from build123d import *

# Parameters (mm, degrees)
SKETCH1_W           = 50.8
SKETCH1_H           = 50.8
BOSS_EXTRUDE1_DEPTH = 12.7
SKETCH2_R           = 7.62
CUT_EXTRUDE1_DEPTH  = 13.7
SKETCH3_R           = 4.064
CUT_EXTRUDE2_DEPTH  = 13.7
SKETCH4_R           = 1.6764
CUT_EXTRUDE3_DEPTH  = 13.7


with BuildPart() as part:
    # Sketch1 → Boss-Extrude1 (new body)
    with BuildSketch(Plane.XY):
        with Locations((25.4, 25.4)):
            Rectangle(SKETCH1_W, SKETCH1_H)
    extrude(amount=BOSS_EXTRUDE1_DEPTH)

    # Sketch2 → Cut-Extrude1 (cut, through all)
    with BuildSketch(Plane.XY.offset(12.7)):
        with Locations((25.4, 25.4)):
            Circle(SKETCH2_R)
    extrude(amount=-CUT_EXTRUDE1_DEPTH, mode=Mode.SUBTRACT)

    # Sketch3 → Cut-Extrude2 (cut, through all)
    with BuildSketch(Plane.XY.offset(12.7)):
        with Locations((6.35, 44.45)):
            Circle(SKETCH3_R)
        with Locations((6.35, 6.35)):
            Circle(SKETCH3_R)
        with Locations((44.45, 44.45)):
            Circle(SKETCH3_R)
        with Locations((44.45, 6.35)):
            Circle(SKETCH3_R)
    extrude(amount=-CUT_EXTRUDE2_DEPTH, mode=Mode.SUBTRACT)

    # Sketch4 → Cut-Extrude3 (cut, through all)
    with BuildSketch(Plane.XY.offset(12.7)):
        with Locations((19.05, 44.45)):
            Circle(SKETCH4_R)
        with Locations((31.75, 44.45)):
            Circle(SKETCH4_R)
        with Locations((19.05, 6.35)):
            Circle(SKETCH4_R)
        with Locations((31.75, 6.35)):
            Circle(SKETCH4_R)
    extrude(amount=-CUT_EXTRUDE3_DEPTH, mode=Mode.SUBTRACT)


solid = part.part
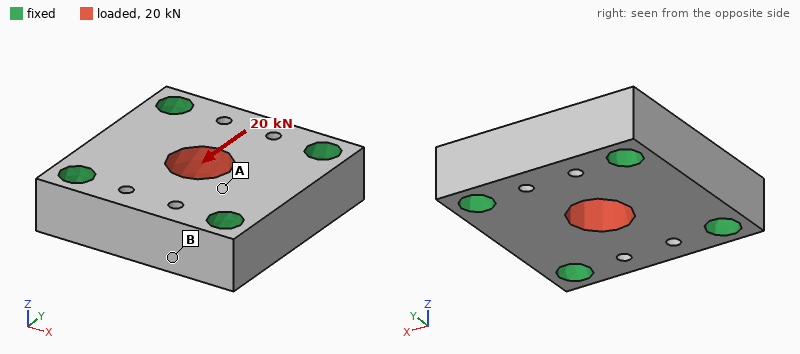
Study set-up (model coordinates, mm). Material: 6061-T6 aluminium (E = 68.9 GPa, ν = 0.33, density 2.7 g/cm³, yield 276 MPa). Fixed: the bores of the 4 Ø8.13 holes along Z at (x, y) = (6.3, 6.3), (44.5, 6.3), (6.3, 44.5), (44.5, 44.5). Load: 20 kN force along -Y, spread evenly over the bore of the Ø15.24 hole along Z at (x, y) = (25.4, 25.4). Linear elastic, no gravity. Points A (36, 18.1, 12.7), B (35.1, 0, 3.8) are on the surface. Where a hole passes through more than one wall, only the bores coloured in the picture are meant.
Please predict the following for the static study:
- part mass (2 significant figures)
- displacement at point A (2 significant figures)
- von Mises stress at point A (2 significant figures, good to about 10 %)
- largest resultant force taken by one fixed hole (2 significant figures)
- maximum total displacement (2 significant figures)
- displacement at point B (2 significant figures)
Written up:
74 g
5.7 µm
30 MPa
5.6 kN
12 µm
4.9 µm
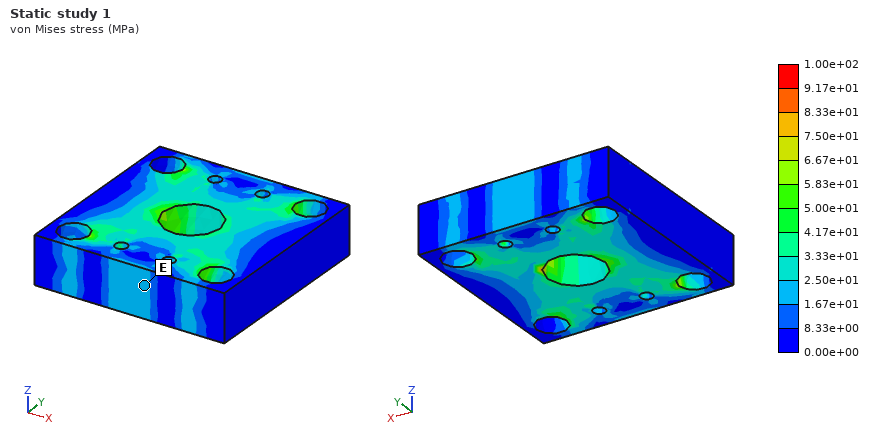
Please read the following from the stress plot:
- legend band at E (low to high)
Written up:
1.67e+01 to 2.50e+01 MPa
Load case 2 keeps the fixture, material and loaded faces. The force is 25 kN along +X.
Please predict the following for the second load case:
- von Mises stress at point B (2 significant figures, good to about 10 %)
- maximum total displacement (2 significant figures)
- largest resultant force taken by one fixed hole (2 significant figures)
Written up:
6.1 MPa
15 µm
6.9 kN
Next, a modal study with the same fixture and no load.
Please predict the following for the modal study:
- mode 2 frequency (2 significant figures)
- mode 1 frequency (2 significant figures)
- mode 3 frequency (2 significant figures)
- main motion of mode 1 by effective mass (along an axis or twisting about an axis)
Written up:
36 kHz
28 kHz
36 kHz
along Z
